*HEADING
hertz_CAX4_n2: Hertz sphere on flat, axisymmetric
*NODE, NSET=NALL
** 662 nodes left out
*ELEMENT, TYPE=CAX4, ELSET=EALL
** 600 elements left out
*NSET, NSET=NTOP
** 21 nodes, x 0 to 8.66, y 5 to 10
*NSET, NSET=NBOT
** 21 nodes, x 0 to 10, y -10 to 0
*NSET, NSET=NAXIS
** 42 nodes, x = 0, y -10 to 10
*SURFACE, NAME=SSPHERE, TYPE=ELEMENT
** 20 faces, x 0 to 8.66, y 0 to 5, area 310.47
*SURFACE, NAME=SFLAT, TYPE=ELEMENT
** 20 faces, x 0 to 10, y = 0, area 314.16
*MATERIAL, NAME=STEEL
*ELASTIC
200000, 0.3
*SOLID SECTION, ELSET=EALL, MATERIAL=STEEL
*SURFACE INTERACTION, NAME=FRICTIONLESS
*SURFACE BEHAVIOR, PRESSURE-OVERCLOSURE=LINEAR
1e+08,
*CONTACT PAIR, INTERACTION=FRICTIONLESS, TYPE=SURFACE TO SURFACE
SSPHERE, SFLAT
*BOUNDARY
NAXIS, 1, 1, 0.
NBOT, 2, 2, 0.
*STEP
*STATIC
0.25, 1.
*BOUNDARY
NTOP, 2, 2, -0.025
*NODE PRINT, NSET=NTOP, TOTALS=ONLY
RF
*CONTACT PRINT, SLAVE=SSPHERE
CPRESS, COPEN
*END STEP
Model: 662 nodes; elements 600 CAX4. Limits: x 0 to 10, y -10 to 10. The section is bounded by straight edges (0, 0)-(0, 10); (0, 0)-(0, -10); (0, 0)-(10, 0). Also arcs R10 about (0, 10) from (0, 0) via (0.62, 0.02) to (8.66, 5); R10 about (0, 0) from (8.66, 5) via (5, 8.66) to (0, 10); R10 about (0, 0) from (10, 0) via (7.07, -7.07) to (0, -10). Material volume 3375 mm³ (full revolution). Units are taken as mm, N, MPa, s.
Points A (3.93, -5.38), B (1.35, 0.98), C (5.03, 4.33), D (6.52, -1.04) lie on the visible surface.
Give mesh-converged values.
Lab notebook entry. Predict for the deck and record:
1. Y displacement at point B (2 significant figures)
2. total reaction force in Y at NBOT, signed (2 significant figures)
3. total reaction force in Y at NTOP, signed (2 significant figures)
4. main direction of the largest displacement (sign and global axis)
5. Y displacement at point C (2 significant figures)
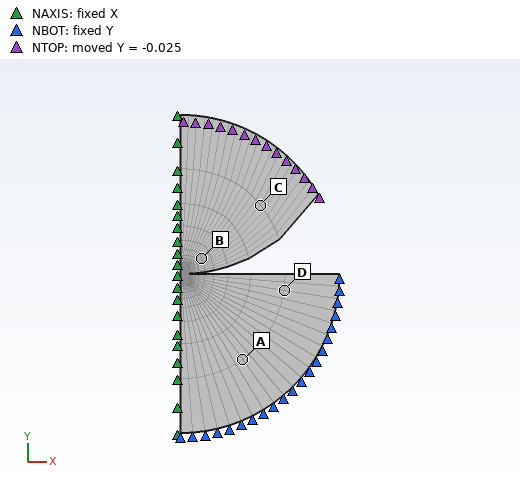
-0.023 mm
1900 N
-1900 N
-Y
-0.025 mm
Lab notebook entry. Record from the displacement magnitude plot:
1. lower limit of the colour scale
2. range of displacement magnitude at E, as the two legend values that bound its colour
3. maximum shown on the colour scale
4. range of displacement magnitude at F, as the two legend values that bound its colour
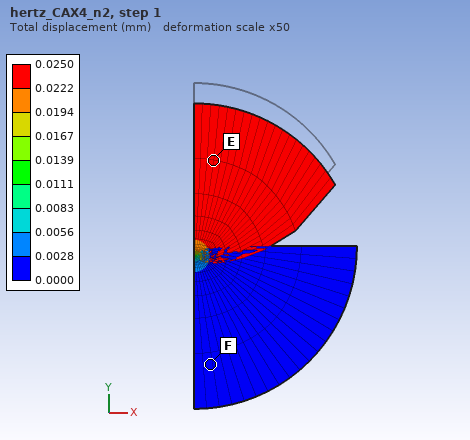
0.0000 mm
0.0222 to 0.0250 mm
0.0250 mm
0.0000 to 0.0028 mm
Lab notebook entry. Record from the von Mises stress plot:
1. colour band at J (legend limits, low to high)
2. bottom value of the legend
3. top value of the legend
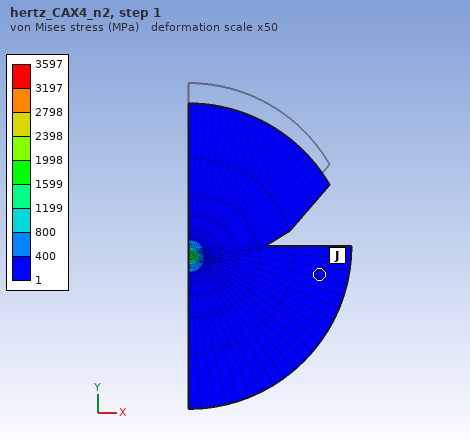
1 to 400 MPa
1 MPa
3597 MPa
